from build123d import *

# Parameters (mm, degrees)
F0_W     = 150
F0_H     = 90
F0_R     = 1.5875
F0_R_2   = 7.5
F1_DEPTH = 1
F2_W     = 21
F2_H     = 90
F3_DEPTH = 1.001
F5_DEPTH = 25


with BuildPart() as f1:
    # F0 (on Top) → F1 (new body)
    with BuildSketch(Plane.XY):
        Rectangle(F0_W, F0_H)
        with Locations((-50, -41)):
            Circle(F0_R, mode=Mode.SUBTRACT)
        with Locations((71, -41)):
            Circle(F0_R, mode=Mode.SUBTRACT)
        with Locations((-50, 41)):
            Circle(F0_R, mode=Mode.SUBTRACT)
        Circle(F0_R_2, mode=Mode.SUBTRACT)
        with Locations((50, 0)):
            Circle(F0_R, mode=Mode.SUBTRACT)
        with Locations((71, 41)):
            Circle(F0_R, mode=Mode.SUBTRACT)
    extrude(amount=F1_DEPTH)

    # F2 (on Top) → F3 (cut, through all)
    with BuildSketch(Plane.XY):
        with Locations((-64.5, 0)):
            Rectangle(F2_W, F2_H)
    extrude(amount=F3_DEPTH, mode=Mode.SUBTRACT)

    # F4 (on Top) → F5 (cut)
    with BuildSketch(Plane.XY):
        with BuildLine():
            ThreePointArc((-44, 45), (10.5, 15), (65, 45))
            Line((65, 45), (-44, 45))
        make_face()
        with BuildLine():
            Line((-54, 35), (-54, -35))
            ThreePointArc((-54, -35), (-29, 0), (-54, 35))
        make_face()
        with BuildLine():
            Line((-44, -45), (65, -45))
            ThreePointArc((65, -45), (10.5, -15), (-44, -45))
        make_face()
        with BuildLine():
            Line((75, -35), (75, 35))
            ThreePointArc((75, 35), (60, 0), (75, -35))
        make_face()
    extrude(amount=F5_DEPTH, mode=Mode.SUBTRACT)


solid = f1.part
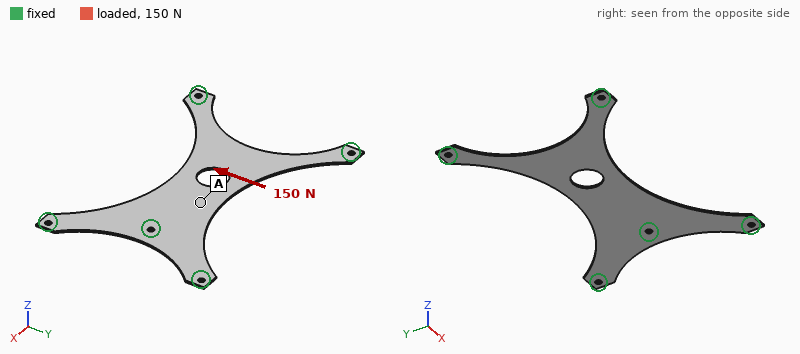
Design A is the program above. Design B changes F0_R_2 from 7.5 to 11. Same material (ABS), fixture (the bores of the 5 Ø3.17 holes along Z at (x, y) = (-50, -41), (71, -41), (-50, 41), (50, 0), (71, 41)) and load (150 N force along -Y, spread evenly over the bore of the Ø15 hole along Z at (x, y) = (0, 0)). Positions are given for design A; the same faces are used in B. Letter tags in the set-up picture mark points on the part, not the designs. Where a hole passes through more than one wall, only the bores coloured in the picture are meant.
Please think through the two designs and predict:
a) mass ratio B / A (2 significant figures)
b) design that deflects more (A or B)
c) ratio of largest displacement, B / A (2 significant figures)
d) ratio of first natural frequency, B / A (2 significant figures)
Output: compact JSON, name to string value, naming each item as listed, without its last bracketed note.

{"mass ratio B / A": "0.96", "design that deflects more": "B", "ratio of largest displacement, B / A": "1.2", "ratio of first natural frequency, B / A": "1.0"}
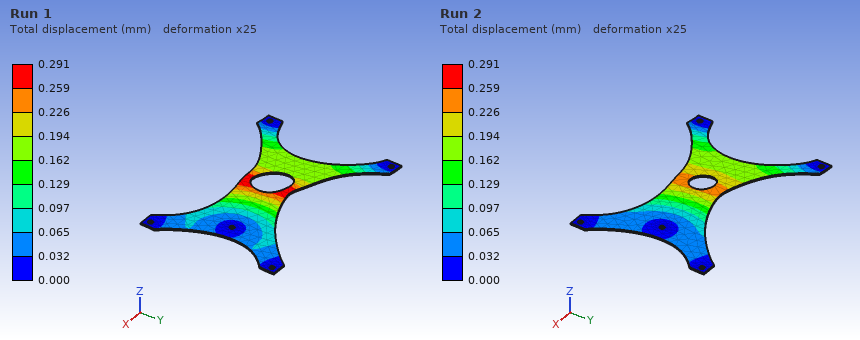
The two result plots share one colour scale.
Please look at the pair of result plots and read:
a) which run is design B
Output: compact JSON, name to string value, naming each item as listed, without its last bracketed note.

{"which run is design B": "Run 1"}
